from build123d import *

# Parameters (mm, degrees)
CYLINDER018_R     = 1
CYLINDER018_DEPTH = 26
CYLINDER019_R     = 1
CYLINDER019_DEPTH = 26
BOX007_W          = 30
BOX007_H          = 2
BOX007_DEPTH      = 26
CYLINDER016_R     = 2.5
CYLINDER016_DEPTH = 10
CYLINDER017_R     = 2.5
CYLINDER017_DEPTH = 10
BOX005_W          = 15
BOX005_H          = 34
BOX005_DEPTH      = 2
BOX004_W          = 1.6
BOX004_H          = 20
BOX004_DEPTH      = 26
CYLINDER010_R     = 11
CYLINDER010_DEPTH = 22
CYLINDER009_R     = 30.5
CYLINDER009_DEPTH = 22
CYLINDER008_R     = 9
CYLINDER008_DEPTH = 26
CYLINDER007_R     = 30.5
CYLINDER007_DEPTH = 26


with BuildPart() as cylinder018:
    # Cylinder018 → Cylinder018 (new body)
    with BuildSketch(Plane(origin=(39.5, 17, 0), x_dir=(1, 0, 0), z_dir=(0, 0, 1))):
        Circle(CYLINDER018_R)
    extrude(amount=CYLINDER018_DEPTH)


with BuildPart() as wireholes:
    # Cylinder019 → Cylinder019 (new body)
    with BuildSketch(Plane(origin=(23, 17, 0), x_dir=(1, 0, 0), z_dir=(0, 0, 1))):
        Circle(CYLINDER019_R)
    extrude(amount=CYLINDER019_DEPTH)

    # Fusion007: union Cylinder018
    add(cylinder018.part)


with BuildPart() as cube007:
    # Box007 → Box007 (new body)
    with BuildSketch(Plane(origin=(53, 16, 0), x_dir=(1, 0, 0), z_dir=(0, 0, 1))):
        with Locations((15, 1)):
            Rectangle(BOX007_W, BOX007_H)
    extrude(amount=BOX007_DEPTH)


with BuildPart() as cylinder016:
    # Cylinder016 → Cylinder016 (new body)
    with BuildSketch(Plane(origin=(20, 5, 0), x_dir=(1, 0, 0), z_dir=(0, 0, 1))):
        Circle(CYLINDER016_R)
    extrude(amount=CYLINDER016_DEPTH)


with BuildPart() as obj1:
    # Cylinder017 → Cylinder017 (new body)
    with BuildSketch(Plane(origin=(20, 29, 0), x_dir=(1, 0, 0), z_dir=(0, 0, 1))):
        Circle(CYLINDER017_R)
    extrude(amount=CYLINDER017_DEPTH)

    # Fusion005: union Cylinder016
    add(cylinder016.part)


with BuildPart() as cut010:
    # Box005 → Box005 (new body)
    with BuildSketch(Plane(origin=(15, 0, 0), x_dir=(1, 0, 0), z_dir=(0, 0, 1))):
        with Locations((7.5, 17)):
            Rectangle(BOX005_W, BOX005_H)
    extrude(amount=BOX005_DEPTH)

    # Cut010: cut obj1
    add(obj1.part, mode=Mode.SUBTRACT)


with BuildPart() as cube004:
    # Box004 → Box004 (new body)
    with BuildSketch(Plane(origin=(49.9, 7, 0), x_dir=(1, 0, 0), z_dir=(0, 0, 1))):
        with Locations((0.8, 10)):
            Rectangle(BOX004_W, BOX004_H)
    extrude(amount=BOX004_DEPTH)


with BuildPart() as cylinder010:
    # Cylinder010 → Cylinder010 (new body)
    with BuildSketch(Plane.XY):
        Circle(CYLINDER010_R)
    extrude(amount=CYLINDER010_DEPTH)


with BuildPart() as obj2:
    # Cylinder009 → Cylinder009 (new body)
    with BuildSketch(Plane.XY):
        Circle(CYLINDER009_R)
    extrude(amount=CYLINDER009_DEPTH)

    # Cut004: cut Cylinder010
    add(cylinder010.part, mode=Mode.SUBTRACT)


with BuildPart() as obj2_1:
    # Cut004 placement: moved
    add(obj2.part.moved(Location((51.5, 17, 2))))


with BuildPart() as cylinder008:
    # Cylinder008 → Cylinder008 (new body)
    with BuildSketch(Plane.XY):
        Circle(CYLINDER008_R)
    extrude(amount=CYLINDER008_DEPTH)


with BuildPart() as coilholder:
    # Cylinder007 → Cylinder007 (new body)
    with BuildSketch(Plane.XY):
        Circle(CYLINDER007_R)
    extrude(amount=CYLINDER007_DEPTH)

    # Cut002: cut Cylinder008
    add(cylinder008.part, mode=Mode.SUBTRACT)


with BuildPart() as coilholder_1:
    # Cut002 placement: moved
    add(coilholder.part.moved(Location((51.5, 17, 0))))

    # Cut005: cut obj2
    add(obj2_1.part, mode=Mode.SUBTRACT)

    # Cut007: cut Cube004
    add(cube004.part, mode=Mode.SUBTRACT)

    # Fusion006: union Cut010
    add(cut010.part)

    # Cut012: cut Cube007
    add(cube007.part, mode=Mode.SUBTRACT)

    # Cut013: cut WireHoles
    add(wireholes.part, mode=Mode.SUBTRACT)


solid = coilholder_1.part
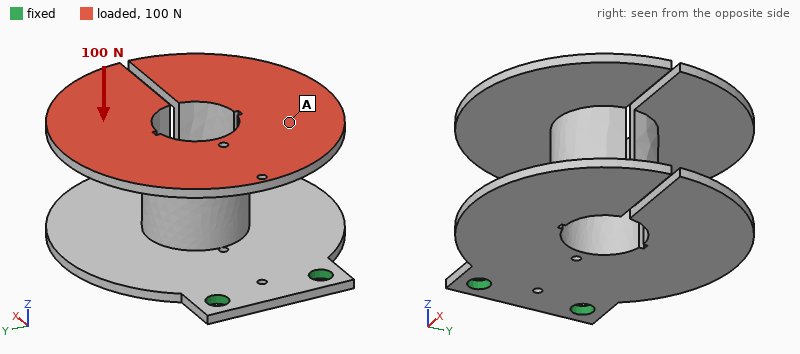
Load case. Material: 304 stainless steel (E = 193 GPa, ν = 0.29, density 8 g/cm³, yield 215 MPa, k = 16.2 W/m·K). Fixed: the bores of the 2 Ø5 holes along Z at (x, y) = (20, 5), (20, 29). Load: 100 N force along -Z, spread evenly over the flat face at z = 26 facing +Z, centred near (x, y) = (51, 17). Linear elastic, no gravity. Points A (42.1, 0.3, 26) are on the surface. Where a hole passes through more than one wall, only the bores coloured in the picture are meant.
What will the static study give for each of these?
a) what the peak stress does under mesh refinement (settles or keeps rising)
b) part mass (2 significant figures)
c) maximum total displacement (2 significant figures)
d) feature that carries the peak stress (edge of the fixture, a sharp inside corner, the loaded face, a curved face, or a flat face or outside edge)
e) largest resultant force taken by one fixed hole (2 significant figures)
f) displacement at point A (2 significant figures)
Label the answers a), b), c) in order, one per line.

a) keeps rising
b) 110 g
c) 0.49 mm
d) edge of the fixture
e) 50 N
f) 0.23 mm
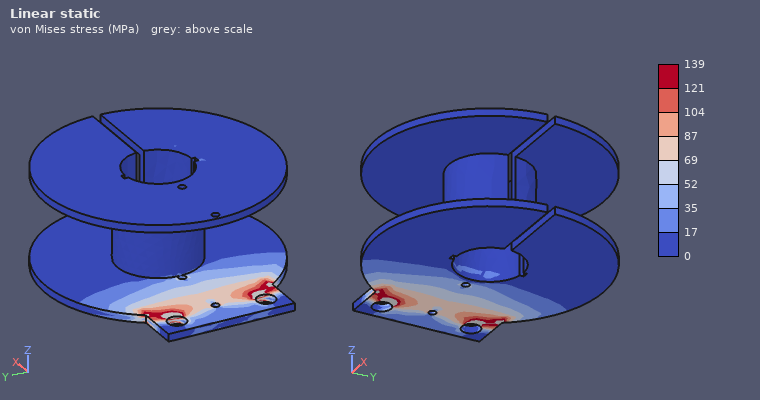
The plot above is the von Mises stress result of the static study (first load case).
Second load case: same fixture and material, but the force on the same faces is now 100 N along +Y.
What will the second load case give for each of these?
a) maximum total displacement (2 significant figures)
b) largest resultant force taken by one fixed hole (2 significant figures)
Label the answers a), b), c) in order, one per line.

a) 0.15 mm
b) 160 N
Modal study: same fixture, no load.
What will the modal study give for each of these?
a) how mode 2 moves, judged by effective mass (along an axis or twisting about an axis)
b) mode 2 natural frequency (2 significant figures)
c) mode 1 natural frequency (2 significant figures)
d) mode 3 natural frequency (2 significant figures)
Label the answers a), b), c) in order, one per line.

a) along Y
b) 600 Hz
c) 250 Hz
d) 770 Hz
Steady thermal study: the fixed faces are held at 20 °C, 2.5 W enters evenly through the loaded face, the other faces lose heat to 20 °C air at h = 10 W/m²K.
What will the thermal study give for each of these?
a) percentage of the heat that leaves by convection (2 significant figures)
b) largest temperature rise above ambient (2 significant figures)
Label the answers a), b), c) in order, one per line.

a) 80 %
b) 32 K
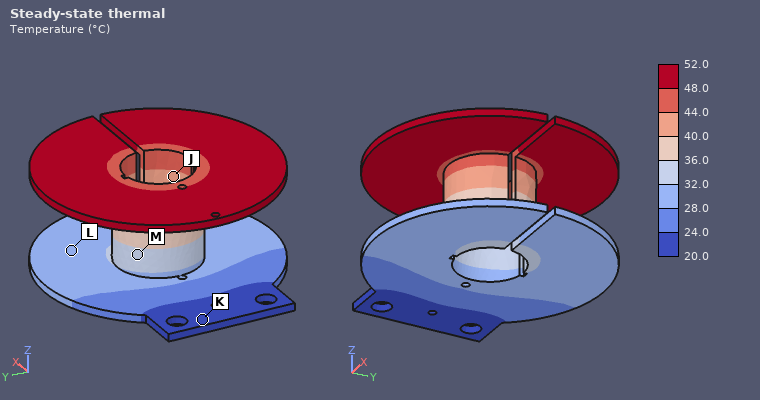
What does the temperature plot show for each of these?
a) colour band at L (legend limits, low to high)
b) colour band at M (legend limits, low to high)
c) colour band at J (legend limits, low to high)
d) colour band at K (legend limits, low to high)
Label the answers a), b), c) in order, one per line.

a) 28.0 to 32.0 °C
b) 32.0 to 36.0 °C
c) 40.0 to 44.0 °C
d) 20.0 to 24.0 °C
